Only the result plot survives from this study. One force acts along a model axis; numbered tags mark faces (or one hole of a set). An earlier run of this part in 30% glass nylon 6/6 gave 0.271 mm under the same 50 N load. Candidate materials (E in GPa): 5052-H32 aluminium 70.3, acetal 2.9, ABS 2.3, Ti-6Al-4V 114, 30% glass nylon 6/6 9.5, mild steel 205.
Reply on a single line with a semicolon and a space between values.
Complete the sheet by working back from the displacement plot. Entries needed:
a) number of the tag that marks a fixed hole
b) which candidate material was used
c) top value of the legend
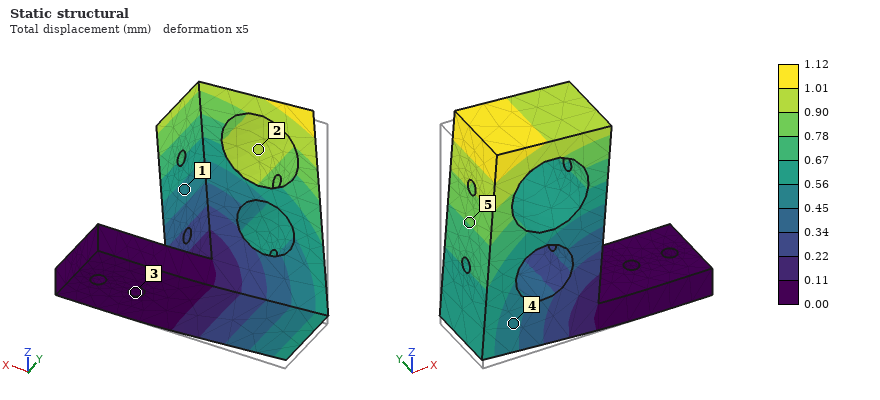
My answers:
3; ABS; 1.12 mm
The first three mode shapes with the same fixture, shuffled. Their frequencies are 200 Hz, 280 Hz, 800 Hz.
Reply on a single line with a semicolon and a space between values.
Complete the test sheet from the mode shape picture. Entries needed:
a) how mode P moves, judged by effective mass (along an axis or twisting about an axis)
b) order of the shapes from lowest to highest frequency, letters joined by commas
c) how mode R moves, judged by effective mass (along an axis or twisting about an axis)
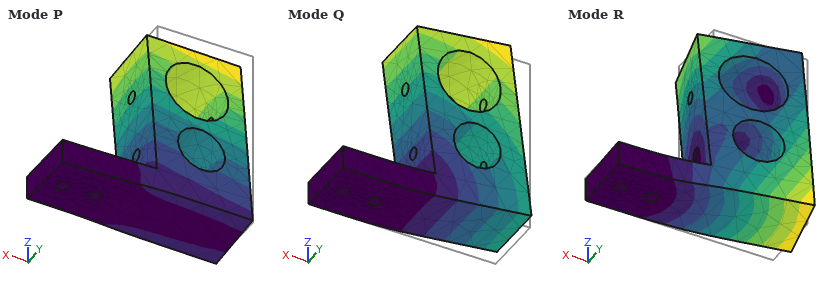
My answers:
along Y; Q, P, R; along Y
